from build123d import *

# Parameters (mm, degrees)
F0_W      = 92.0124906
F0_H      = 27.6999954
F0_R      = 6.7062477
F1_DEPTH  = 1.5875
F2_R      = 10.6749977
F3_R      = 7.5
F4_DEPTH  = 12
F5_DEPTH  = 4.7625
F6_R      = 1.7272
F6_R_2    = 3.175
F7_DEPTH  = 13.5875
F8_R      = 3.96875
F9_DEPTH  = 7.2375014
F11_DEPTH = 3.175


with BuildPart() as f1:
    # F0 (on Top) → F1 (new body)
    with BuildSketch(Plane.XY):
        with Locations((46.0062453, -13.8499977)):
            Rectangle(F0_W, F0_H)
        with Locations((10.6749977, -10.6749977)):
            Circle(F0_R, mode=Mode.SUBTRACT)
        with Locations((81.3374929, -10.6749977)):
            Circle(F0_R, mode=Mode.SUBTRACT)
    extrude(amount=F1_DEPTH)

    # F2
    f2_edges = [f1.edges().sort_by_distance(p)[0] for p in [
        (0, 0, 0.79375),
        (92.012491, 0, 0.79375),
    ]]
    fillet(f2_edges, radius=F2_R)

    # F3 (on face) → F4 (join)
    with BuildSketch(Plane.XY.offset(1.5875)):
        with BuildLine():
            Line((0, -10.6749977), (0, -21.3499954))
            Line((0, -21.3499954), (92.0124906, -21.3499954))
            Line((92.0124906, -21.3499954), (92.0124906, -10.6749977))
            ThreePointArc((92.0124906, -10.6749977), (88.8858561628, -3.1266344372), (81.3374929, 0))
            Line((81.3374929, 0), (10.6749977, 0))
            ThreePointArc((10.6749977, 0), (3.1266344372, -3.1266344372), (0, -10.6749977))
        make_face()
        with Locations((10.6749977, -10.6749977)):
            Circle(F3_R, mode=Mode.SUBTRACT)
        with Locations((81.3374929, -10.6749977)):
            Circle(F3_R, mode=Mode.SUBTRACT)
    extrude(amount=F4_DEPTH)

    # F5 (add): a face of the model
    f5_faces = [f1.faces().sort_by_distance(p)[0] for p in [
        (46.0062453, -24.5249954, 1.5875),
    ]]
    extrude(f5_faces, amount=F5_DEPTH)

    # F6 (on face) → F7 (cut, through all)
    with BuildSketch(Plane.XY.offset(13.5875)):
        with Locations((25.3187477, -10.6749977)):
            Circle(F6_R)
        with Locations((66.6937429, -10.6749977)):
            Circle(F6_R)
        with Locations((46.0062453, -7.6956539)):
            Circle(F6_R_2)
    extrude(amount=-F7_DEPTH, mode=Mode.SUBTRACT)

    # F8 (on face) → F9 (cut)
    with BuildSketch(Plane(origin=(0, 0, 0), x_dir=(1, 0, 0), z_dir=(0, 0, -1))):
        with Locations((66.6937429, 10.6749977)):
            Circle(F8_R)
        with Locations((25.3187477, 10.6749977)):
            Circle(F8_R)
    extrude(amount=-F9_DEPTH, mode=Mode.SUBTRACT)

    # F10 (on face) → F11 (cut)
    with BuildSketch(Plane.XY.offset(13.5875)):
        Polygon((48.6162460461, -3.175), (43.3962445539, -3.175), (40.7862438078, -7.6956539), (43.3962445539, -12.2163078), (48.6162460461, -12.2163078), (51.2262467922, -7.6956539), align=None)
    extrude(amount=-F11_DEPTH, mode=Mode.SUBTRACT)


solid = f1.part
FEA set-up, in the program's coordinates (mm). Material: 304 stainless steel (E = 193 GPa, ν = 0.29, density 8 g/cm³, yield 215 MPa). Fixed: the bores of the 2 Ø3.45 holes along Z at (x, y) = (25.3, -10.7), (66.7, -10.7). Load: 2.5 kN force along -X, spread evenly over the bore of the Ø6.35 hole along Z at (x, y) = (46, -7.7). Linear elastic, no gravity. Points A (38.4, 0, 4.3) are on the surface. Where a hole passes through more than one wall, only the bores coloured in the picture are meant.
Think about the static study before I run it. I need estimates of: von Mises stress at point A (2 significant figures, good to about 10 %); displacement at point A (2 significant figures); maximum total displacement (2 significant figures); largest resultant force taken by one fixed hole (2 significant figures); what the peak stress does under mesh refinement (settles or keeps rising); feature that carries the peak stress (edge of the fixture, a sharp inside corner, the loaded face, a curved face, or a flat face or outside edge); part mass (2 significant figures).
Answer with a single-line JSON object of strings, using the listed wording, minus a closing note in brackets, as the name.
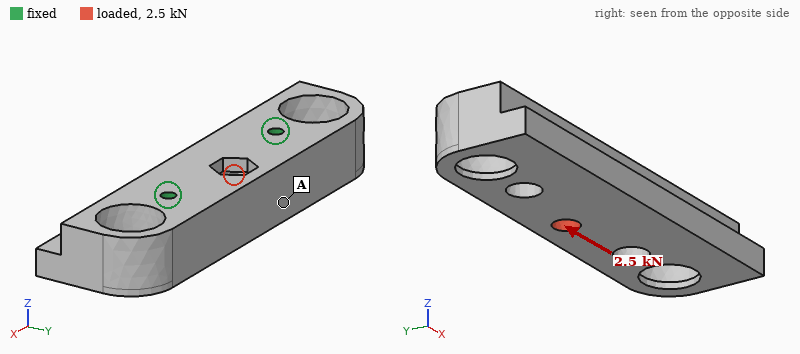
{"von Mises stress at point A": "4.0 MPa", "displacement at point A": "0.99 µm", "maximum total displacement": "1.4 µm", "largest resultant force taken by one fixed hole": "1.3 kN", "what the peak stress does under mesh refinement": "keeps rising", "feature that carries the peak stress": "edge of the fixture", "part mass": "190 g"}
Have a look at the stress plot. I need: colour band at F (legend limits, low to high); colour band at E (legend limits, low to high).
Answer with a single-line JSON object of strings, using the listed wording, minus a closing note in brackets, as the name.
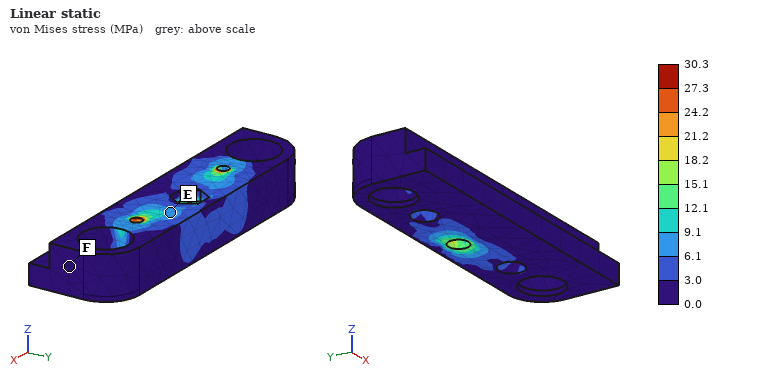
{"colour band at F": "0.0 to 3.0 MPa", "colour band at E": "6.1 to 9.1 MPa"}
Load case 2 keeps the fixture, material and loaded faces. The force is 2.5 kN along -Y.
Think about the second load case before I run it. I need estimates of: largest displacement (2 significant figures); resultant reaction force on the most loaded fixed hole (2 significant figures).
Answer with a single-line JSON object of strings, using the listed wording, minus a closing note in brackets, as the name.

{"largest displacement": "7.8 µm", "resultant reaction force on the most loaded fixed hole": "1.3 kN"}
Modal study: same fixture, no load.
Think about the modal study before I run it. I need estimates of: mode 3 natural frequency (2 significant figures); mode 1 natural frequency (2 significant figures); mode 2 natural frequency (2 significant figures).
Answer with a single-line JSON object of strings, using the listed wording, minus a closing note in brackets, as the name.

{"mode 3 natural frequency": "9700 Hz", "mode 1 natural frequency": "7300 Hz", "mode 2 natural frequency": "8800 Hz"}
